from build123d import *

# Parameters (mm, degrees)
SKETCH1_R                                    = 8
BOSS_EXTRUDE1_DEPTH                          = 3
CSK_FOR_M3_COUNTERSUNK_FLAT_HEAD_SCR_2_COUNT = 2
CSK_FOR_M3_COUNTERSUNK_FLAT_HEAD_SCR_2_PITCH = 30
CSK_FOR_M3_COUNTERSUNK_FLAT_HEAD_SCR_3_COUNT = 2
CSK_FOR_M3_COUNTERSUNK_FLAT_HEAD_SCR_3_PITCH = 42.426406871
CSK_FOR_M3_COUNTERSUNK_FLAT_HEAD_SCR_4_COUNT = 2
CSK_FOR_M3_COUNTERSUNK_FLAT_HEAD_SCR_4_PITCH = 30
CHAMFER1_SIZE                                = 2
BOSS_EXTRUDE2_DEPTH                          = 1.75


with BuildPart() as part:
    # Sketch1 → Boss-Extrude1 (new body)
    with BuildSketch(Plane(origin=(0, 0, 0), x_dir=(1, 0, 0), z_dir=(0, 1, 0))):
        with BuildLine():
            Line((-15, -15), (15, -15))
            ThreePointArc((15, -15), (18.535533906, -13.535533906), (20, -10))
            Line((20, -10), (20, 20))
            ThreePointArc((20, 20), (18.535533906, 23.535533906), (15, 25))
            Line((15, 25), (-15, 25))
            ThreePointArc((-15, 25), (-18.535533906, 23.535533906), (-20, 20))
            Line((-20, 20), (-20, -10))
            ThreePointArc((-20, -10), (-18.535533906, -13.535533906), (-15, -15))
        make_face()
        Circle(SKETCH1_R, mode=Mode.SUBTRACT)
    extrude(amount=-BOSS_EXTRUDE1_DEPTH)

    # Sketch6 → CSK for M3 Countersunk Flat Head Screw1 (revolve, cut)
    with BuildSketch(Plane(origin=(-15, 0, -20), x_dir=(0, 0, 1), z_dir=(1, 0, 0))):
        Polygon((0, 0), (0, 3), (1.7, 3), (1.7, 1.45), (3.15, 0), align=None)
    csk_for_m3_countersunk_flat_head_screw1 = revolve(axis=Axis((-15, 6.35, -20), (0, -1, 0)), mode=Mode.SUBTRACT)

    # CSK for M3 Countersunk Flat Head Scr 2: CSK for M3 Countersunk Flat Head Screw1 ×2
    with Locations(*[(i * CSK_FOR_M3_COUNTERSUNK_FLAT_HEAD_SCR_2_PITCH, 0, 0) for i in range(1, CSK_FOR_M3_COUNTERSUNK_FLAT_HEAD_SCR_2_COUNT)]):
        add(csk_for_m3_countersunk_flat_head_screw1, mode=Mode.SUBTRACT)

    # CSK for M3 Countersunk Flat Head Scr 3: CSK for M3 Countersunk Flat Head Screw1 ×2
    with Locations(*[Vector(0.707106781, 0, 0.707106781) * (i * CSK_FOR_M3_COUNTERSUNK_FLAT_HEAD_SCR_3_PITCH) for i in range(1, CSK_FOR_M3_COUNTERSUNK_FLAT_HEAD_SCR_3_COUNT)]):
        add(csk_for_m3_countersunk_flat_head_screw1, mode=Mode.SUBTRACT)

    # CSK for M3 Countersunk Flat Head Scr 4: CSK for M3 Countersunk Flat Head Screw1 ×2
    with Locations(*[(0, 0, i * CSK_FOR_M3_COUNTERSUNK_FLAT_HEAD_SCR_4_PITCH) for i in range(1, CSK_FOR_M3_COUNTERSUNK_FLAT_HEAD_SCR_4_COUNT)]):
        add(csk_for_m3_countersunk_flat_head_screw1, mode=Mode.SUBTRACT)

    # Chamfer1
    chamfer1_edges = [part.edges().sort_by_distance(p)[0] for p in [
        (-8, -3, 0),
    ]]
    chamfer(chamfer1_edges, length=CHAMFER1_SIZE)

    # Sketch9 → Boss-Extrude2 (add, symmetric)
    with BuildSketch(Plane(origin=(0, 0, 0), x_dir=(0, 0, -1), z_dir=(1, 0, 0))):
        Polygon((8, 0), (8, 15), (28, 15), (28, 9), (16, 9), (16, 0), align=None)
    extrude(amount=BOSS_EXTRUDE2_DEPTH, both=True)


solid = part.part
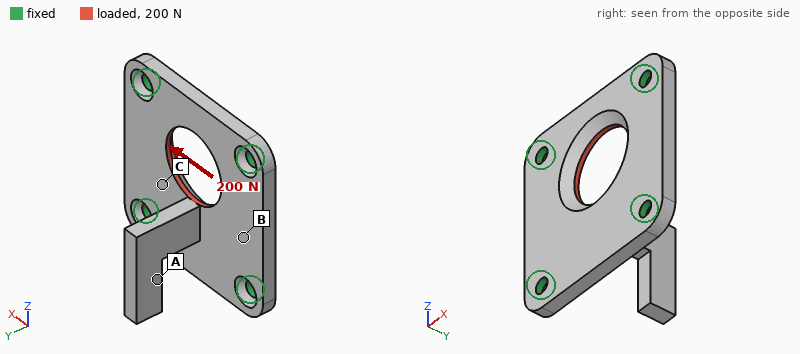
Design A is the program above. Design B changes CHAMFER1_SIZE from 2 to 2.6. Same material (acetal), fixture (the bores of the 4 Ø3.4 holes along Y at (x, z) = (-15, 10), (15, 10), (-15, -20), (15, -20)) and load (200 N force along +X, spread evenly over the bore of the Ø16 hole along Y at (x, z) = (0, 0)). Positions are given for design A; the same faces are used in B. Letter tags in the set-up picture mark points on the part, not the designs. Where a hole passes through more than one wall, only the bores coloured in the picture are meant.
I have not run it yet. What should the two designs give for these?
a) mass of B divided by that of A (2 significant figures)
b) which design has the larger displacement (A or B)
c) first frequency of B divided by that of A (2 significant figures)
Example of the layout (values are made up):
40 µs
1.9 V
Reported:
0.98
B
0.99
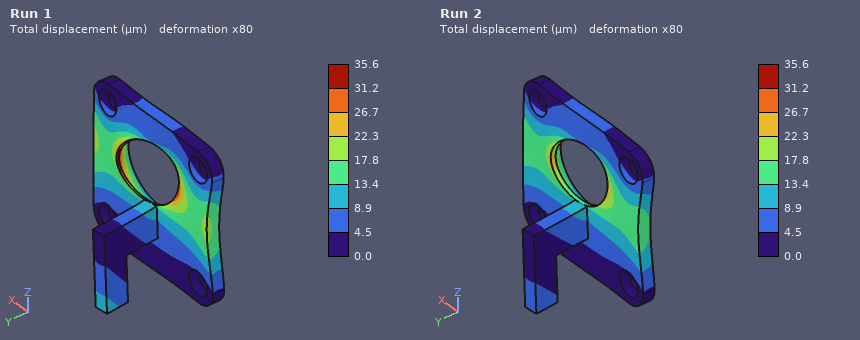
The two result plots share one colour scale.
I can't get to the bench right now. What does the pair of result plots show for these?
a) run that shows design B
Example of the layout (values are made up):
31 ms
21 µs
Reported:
Run 1
